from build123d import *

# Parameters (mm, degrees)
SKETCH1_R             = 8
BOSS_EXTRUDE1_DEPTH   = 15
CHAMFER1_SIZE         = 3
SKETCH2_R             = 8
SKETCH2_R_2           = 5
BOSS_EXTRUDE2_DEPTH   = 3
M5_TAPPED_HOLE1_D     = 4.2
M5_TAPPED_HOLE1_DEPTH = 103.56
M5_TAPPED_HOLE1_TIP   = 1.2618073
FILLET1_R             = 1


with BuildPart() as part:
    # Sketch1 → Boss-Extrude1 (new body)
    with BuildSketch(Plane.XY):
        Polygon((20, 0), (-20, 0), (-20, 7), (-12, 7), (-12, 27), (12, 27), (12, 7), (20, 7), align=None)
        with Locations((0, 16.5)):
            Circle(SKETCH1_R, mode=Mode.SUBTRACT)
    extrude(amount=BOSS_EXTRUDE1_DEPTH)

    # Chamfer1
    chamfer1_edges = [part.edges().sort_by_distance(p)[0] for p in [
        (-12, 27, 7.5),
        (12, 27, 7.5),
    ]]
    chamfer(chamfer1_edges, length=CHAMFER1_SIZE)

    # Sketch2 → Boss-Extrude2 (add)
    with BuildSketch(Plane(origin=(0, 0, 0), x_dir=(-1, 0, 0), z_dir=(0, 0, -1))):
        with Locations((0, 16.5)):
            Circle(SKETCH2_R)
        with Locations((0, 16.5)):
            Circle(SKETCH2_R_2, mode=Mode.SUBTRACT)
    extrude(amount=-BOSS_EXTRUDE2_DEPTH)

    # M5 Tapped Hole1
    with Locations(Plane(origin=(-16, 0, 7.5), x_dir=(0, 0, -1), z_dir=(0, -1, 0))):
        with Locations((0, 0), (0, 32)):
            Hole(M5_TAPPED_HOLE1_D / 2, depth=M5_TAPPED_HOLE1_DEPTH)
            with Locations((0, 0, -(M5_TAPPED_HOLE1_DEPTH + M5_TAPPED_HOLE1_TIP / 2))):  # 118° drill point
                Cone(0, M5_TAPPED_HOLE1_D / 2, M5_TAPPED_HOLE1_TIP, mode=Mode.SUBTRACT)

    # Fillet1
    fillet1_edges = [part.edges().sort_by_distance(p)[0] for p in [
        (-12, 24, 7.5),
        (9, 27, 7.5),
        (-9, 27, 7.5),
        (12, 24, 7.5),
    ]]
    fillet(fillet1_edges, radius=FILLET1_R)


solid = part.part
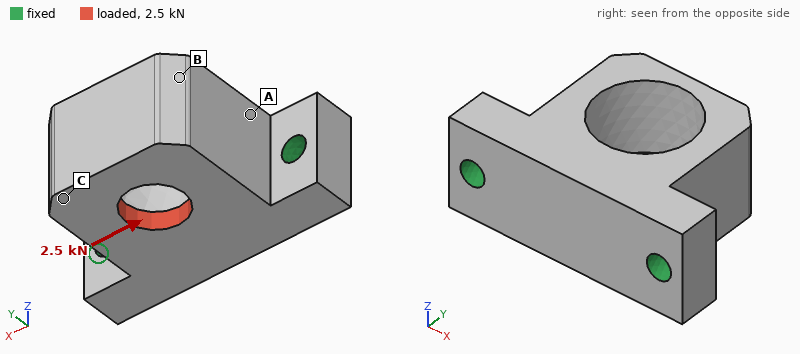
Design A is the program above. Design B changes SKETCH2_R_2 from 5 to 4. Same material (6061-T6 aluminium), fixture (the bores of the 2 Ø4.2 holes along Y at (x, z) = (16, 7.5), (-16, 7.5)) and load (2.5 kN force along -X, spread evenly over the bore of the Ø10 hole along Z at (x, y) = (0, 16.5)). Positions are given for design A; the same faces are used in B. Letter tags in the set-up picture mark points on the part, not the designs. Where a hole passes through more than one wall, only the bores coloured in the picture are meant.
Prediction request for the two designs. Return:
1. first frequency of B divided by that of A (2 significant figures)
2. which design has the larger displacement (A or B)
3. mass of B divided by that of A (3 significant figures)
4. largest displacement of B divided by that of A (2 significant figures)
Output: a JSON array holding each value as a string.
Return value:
["0.99", "A", "1.01", "0.87"]
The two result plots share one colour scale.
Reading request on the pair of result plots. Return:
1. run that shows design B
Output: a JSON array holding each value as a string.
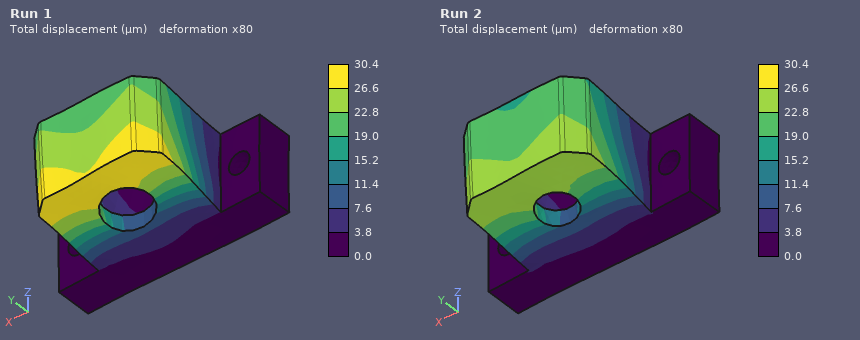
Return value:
["Run 2"]
